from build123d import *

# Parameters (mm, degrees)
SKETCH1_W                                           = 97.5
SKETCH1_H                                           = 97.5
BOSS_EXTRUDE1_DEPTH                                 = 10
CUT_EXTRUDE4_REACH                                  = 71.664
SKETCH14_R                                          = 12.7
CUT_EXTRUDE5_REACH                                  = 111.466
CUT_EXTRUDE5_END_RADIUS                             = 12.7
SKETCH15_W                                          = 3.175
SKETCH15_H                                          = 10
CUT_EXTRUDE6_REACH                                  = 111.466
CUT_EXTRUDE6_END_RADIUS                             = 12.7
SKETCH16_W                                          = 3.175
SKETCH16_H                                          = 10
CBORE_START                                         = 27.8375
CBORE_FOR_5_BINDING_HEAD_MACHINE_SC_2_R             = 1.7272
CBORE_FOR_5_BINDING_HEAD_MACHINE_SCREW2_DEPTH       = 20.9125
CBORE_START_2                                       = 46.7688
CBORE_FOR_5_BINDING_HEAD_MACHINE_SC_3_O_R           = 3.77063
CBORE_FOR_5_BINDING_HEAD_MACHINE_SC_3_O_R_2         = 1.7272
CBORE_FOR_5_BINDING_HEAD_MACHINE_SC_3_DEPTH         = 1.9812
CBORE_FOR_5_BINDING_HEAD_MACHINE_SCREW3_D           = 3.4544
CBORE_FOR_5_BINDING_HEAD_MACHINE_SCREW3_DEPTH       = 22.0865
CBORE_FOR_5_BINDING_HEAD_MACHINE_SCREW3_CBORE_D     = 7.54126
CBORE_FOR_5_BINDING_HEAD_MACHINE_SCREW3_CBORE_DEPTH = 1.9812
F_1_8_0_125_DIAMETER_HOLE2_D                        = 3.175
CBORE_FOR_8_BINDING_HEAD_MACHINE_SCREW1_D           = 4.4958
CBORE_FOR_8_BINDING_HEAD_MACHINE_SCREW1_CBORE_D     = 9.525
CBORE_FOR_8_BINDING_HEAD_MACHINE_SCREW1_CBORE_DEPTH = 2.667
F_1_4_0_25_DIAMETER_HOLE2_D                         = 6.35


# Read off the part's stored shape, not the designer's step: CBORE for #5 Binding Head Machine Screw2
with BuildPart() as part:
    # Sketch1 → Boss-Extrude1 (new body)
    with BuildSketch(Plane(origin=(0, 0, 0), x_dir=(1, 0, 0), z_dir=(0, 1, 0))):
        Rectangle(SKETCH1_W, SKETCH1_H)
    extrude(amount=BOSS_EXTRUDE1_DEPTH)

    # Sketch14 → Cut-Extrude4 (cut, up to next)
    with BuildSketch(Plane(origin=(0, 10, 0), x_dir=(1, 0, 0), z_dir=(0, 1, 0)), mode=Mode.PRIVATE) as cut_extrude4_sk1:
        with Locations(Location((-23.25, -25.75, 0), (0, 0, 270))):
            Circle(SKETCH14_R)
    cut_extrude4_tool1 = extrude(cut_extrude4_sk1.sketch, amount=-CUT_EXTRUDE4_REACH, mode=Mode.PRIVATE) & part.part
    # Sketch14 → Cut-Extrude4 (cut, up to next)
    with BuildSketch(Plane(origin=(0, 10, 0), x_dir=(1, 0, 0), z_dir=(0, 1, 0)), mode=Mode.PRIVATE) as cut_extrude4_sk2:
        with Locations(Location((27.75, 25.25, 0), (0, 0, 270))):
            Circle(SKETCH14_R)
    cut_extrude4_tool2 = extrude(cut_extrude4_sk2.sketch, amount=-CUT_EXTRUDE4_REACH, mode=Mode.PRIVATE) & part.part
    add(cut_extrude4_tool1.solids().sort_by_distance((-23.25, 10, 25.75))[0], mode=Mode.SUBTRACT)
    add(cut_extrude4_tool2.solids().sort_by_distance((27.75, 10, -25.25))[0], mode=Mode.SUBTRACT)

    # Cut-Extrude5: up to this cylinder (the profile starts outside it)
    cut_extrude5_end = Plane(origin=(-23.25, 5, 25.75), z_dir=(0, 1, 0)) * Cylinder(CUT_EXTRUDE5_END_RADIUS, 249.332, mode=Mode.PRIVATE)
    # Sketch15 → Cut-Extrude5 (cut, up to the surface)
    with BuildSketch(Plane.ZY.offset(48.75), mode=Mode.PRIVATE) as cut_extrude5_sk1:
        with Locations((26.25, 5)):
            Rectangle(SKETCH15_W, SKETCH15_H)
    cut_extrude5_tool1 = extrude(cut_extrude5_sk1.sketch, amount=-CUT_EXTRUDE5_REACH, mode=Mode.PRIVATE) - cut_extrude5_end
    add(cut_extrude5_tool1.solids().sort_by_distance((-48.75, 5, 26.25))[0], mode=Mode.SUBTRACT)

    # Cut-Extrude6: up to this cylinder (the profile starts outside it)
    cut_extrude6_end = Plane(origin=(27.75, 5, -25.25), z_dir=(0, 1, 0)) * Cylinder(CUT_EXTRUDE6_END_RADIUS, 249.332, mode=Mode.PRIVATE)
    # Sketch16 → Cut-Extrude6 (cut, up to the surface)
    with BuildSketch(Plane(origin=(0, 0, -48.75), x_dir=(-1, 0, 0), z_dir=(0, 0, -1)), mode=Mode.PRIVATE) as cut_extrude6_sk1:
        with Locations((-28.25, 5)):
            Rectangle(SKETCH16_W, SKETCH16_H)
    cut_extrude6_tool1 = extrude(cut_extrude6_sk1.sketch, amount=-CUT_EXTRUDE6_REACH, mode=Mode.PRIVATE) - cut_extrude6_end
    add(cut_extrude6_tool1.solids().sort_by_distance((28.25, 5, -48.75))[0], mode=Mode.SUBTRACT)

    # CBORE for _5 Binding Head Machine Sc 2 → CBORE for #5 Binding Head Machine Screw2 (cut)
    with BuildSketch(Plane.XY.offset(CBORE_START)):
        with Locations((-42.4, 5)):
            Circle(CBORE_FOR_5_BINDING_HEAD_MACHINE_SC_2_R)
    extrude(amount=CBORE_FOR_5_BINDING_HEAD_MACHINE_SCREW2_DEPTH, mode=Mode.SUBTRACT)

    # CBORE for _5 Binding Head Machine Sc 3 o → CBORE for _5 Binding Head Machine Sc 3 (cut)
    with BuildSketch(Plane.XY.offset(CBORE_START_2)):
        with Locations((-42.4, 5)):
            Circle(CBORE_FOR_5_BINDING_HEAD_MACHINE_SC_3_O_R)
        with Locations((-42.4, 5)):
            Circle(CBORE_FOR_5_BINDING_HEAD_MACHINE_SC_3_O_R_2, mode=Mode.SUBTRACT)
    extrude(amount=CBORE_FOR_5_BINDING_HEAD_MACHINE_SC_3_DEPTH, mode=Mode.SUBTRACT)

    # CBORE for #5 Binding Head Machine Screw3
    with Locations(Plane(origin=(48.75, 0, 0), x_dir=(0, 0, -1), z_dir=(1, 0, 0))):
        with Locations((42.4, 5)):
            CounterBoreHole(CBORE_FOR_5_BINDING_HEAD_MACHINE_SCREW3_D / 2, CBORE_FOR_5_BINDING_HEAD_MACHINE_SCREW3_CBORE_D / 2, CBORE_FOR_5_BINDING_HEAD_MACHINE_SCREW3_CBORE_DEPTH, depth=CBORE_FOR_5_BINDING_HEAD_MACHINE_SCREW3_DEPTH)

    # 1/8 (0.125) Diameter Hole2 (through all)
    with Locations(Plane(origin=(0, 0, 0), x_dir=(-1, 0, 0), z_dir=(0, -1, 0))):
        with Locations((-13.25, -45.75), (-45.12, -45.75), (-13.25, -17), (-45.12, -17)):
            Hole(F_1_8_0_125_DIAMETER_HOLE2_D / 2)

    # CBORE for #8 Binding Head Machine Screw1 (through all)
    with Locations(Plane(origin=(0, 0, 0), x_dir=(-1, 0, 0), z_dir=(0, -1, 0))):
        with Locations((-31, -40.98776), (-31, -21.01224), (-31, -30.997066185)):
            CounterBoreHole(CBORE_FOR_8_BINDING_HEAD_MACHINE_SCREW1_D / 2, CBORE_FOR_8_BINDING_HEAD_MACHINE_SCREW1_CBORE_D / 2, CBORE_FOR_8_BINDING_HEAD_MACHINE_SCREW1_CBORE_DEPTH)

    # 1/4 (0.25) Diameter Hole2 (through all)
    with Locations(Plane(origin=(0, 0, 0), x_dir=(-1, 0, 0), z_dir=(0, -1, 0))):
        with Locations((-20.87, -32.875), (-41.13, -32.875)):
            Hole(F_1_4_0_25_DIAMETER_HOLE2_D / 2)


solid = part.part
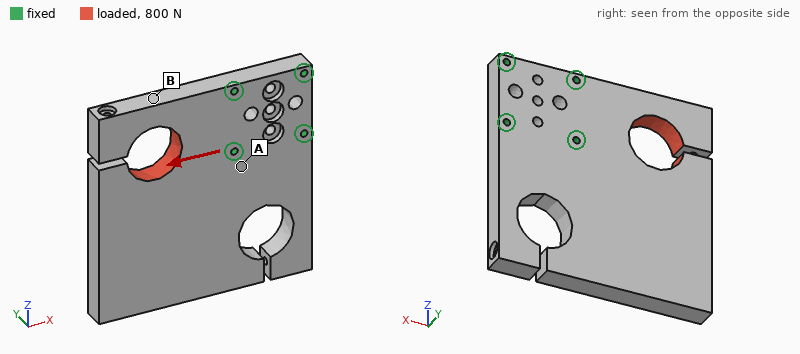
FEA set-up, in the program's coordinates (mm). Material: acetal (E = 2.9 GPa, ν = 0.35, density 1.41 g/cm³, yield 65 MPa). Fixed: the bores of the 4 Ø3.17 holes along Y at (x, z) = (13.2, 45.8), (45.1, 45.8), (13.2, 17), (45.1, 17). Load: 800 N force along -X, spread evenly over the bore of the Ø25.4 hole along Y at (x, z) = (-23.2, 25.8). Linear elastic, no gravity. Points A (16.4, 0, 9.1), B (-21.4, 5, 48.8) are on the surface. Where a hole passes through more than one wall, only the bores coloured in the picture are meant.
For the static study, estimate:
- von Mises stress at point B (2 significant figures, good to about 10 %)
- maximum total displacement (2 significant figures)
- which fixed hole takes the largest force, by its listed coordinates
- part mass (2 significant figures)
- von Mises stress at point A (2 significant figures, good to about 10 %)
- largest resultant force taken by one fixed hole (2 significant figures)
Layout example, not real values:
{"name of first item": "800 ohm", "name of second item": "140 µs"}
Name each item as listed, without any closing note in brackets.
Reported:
{"von Mises stress at point B": "6.5 MPa", "maximum total displacement": "0.40 mm", "which fixed hole takes the largest force, by its listed coordinates": "(13.2, 17)", "part mass": "120 g", "von Mises stress at point A": "1.4 MPa", "largest resultant force taken by one fixed hole": "450 N"}
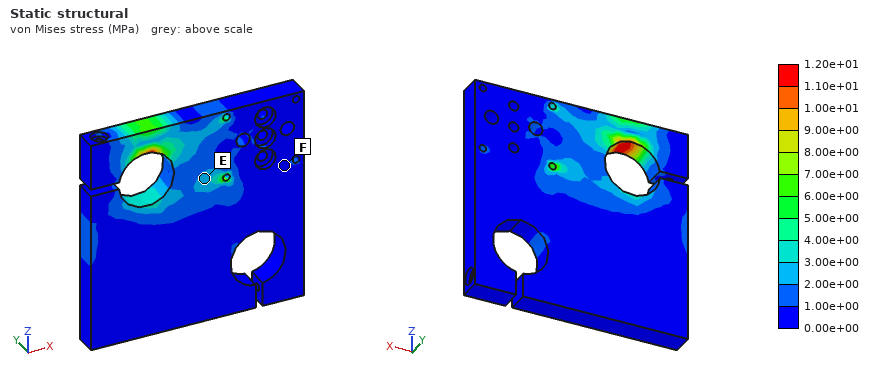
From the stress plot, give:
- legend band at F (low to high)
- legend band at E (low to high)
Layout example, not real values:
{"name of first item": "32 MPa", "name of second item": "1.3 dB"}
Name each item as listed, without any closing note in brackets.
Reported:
{"legend band at F": "0.00e+00 to 1.00e+00 MPa", "legend band at E": "2.00e+00 to 3.00e+00 MPa"}
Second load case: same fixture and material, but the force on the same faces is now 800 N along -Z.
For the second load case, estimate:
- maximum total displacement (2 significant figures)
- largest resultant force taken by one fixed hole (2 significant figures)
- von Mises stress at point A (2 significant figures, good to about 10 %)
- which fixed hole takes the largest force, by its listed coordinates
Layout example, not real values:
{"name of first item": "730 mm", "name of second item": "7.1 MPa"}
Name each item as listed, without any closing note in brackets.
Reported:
{"maximum total displacement": "0.69 mm", "largest resultant force taken by one fixed hole": "890 N", "von Mises stress at point A": "3.0 MPa", "which fixed hole takes the largest force, by its listed coordinates": "(13.2, 17)"}
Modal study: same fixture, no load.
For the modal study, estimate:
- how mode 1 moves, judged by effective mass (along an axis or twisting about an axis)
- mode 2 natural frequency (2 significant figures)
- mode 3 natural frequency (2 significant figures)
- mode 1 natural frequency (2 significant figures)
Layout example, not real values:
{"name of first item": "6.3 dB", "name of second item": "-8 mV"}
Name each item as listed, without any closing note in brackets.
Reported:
{"how mode 1 moves, judged by effective mass": "along Y", "mode 2 natural frequency": "540 Hz", "mode 3 natural frequency": "690 Hz", "mode 1 natural frequency": "310 Hz"}
